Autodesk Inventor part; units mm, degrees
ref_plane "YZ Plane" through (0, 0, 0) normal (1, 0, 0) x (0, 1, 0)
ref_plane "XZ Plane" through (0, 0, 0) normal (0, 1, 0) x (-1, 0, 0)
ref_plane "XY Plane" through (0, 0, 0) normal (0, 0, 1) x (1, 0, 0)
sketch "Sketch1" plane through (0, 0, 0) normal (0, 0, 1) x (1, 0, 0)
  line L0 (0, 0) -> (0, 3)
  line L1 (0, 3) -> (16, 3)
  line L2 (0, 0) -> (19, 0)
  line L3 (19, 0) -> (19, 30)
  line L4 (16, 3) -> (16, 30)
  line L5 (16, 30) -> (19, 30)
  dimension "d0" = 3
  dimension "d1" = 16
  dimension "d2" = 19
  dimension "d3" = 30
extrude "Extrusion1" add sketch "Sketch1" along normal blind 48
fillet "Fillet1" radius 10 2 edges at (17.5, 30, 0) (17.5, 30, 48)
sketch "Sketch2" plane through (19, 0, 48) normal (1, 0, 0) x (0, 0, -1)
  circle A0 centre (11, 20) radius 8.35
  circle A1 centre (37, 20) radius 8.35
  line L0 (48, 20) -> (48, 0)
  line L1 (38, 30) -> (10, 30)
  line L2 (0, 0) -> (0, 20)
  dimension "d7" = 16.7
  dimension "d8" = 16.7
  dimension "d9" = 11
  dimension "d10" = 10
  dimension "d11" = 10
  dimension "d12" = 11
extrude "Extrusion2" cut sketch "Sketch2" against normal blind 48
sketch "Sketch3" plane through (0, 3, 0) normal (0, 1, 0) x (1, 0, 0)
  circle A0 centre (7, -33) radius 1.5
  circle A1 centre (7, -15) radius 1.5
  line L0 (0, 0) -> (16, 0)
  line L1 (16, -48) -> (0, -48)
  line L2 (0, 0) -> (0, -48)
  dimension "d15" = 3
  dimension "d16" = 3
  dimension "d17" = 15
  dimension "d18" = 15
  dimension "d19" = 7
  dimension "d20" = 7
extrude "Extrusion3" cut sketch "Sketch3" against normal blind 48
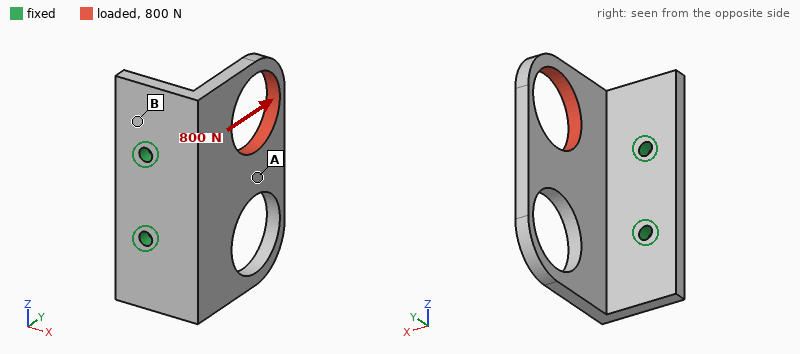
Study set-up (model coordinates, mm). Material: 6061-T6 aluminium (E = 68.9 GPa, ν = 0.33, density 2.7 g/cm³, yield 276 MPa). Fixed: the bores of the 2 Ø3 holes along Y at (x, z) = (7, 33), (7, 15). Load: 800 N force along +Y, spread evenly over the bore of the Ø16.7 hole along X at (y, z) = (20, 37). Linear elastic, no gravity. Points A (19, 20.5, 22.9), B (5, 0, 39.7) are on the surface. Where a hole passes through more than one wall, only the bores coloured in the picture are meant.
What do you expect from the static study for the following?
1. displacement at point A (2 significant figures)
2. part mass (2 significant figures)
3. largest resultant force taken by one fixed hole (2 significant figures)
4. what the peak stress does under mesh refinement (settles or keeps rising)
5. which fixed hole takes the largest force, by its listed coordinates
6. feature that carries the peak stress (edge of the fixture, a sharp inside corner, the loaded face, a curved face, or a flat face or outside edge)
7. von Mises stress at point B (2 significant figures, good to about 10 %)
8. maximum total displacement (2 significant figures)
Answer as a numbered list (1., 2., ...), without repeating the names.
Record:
1. 0.17 mm
2. 14 g
3. 840 N
4. keeps rising
5. (7, 33)
6. edge of the fixture
7. 79 MPa
8. 0.33 mm
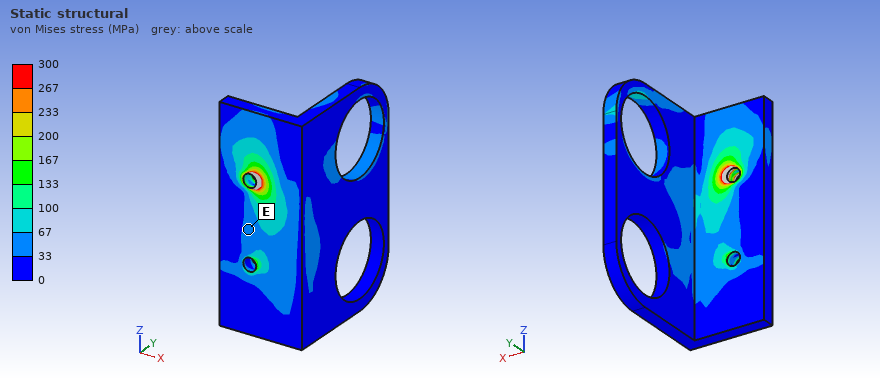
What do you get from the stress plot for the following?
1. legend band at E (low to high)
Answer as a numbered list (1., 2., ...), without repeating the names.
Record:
1. 33 to 67 MPa
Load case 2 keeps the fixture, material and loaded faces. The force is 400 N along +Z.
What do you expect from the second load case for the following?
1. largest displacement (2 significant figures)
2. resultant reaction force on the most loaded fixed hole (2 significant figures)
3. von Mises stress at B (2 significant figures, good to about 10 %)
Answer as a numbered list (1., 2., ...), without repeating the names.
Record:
1. 0.12 mm
2. 430 N
3. 34 MPa
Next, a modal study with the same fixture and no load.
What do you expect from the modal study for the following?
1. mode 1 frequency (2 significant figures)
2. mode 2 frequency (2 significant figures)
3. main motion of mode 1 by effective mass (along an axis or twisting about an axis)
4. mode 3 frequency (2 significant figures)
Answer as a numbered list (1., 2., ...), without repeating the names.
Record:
1. 2500 Hz
2. 4200 Hz
3. along X
4. 6300 Hz
